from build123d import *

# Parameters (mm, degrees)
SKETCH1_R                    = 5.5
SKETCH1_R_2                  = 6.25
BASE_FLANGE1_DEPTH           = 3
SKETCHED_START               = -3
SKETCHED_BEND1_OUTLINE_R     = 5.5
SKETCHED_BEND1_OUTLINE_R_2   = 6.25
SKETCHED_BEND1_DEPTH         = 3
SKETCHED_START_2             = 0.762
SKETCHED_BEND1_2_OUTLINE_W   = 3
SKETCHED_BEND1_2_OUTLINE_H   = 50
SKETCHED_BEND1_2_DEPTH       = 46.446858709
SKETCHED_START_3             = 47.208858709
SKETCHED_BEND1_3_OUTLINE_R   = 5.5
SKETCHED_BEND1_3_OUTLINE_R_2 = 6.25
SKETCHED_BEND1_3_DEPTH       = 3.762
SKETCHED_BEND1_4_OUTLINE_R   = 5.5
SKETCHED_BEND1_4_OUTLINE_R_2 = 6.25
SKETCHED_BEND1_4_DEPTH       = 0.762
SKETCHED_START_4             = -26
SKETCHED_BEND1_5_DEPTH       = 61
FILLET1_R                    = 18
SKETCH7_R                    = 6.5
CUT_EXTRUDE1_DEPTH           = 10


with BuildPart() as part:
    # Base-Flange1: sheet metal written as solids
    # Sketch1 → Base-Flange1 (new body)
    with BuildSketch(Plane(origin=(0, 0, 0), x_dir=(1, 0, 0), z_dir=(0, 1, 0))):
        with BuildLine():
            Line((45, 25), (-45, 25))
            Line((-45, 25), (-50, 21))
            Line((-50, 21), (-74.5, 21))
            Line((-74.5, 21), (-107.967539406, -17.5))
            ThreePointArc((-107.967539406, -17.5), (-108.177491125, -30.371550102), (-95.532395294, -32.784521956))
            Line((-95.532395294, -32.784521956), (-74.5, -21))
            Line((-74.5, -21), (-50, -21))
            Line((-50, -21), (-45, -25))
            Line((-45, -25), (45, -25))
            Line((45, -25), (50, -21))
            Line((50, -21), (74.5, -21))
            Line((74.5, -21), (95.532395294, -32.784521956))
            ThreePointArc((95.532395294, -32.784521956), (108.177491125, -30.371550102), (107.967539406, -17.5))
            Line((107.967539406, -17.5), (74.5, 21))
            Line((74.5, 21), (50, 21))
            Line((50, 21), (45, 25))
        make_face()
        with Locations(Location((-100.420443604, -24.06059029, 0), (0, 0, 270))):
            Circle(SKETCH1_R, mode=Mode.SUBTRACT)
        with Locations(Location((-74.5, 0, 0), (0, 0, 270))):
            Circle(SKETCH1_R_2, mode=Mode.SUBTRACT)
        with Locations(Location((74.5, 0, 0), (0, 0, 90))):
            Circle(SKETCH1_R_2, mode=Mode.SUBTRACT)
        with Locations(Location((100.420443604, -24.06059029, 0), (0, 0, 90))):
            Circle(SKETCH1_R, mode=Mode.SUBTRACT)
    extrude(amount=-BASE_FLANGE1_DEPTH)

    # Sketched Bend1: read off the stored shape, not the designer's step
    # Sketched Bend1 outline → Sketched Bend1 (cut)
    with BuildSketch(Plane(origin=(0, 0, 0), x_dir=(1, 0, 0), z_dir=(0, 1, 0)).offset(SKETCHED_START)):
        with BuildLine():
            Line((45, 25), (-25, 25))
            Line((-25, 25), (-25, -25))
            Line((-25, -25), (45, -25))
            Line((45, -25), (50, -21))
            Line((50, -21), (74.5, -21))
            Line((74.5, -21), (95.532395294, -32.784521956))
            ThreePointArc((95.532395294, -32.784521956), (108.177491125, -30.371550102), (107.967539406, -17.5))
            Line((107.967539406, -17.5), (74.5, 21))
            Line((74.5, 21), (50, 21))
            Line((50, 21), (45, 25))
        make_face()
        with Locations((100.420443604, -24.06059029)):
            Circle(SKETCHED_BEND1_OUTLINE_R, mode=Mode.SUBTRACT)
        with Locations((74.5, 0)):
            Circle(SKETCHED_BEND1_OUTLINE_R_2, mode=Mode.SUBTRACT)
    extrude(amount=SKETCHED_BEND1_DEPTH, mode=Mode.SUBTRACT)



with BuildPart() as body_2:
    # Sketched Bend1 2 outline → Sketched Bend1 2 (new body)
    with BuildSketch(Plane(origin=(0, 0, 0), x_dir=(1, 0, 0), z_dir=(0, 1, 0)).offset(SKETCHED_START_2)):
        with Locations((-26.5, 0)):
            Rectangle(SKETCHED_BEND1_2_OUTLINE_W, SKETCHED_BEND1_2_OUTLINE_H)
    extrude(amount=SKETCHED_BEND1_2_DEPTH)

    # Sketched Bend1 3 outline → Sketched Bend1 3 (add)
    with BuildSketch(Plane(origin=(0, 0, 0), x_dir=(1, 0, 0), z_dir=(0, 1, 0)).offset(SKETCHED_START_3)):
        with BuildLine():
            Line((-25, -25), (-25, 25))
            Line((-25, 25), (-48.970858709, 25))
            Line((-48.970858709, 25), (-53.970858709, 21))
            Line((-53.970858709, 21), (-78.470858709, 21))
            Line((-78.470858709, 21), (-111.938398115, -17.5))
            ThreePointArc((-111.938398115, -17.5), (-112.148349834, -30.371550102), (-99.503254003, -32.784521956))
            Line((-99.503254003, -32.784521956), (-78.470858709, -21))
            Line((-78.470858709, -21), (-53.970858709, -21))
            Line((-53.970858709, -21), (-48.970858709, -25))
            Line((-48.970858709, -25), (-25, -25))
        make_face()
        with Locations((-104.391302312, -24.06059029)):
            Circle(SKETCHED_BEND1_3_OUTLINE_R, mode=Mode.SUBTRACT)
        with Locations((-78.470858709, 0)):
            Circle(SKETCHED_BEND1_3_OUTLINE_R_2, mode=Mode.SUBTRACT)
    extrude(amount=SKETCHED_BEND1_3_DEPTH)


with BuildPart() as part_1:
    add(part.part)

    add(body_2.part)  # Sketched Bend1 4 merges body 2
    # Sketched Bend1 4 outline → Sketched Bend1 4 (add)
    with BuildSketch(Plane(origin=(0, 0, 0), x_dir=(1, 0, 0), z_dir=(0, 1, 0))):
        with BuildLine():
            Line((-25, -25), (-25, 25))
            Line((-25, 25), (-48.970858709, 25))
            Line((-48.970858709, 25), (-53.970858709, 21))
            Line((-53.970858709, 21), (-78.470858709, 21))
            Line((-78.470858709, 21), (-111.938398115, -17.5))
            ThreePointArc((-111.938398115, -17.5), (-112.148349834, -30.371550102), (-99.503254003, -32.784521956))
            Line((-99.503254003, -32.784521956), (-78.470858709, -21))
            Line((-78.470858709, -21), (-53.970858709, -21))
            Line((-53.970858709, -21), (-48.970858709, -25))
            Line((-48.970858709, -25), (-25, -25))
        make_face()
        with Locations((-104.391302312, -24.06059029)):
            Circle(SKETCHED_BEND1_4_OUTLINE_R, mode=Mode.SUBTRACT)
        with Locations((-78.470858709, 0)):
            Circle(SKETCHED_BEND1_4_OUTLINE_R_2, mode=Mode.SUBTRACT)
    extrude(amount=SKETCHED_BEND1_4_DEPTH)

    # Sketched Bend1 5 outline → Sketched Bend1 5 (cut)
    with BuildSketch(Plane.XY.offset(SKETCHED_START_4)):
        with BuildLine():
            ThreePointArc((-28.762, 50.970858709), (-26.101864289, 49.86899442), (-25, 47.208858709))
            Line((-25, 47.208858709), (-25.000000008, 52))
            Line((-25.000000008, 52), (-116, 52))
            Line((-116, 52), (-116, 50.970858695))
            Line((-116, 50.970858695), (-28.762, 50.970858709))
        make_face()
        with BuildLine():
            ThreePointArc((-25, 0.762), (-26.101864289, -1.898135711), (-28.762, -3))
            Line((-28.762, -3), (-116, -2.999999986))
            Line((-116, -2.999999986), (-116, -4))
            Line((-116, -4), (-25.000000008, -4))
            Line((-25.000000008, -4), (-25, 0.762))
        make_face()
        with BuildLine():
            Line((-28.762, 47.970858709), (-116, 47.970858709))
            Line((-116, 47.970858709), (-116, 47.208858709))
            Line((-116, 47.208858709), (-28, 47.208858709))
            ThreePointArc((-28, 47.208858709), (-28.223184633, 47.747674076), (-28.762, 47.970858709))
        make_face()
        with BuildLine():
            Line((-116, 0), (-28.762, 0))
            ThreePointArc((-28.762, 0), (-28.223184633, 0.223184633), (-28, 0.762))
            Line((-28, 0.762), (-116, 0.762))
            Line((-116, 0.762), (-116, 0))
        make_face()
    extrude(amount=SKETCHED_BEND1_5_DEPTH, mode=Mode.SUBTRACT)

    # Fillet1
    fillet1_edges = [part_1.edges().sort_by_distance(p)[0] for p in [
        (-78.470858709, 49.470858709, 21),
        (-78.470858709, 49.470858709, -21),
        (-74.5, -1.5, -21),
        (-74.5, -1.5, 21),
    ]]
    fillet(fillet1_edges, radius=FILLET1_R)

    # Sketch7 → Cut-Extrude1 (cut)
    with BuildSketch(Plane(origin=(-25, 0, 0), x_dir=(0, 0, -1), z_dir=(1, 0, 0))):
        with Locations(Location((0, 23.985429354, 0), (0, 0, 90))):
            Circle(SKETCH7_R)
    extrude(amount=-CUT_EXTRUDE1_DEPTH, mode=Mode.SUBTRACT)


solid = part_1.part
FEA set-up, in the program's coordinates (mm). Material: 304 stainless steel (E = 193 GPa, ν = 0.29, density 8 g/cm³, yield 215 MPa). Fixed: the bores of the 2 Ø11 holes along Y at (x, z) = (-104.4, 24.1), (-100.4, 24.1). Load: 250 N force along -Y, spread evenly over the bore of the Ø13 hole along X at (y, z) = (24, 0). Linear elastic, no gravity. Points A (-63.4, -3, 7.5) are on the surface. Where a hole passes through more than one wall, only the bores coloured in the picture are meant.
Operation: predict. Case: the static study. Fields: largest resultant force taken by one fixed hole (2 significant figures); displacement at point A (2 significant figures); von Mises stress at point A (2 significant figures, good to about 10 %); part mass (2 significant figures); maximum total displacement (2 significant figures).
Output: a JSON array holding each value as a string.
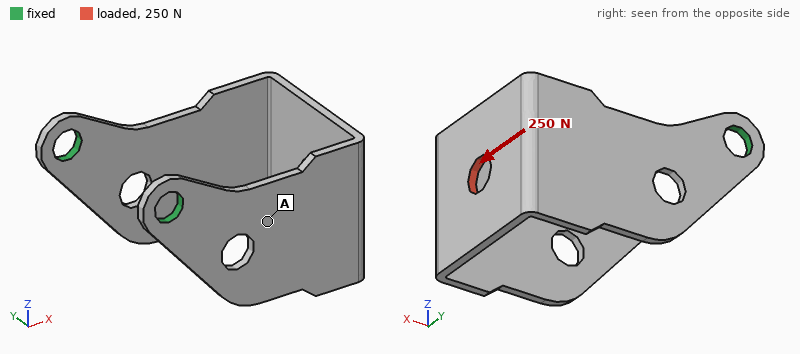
["240 N", "0.17 mm", "15 MPa", "210 g", "0.36 mm"]
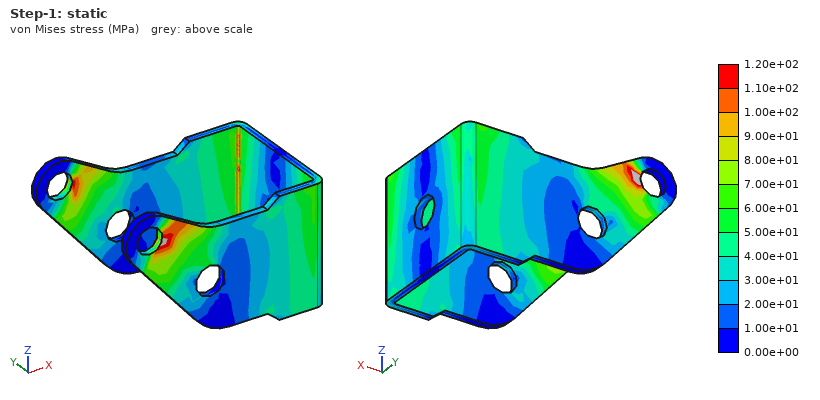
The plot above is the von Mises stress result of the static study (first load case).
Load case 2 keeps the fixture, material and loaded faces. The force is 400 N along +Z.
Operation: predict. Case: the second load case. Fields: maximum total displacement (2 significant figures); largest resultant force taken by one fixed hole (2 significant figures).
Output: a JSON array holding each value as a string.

["62 µm", "200 N"]
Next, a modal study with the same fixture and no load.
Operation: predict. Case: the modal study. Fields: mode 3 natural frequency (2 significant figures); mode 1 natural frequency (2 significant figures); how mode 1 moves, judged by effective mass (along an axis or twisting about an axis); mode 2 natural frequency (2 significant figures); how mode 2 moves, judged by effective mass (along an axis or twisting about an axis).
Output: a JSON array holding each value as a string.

["1400 Hz", "390 Hz", "along Y", "1300 Hz", "along Z"]
